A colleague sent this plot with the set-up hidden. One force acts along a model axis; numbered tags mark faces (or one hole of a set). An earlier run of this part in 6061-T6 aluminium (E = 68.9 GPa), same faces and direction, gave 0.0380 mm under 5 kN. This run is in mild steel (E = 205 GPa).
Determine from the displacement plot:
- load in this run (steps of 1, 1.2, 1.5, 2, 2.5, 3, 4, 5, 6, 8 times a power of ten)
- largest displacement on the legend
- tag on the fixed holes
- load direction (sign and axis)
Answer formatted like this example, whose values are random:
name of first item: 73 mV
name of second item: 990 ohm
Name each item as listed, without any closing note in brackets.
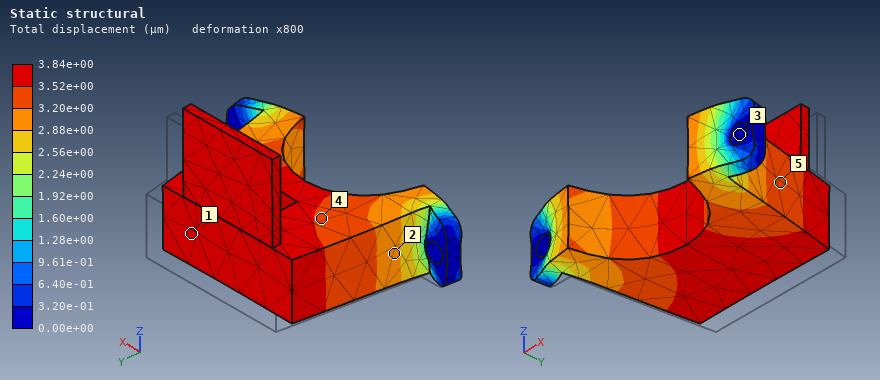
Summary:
load in this run: 1.5 kN
largest displacement on the legend: 3.84e+00 µm
tag on the fixed holes: 3
load direction: -Y
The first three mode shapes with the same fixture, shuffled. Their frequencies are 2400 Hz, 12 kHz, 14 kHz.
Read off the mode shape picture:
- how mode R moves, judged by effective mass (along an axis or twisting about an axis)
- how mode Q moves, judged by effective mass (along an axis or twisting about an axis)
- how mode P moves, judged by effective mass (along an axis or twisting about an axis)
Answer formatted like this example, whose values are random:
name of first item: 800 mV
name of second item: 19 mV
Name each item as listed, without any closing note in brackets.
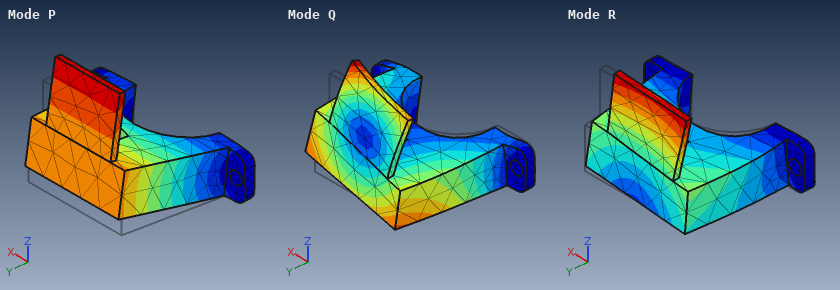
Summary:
how mode R moves, judged by effective mass: along X
how mode Q moves, judged by effective mass: along X
how mode P moves, judged by effective mass: along Z
